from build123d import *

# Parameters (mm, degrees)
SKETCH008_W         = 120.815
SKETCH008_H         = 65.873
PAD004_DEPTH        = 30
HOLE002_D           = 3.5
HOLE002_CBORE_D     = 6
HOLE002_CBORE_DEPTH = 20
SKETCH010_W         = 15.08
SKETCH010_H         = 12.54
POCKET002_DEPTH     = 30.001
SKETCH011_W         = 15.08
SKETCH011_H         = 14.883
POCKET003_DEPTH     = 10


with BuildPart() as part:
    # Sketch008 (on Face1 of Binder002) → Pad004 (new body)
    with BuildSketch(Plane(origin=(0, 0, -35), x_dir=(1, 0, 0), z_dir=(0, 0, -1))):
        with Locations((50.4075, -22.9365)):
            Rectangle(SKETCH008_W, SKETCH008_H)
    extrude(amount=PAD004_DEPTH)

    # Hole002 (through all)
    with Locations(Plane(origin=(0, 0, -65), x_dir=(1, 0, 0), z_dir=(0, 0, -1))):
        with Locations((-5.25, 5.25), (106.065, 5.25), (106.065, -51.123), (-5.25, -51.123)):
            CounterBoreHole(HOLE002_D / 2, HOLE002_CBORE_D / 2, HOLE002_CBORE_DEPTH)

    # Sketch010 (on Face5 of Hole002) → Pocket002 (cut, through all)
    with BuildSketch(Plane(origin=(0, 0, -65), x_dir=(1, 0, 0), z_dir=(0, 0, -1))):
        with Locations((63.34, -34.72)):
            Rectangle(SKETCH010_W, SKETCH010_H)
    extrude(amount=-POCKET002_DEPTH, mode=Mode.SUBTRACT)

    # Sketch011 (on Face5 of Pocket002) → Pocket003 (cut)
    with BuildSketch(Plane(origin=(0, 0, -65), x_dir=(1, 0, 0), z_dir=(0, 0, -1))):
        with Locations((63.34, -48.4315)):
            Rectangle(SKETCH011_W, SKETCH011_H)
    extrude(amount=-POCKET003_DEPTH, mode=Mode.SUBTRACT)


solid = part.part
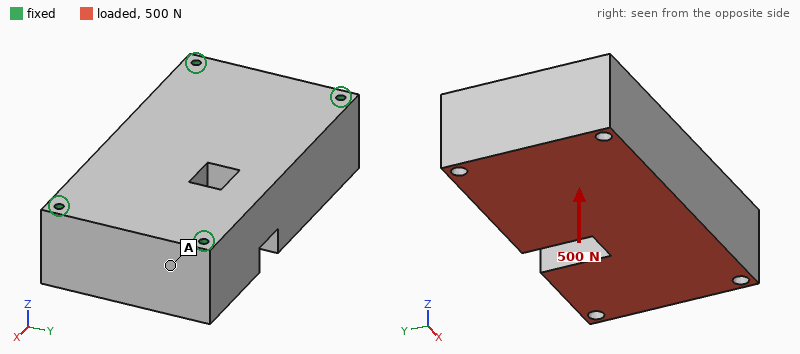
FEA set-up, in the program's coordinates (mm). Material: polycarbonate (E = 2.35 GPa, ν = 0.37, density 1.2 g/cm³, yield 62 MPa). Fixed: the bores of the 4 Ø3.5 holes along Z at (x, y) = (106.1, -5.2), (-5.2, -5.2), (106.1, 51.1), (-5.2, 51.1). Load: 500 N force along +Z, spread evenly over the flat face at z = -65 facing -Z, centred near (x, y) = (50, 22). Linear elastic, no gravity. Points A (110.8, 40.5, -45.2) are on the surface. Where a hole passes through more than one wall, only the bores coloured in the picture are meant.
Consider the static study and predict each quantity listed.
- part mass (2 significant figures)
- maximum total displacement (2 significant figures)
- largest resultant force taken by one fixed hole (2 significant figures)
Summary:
270 g
31 µm
160 N
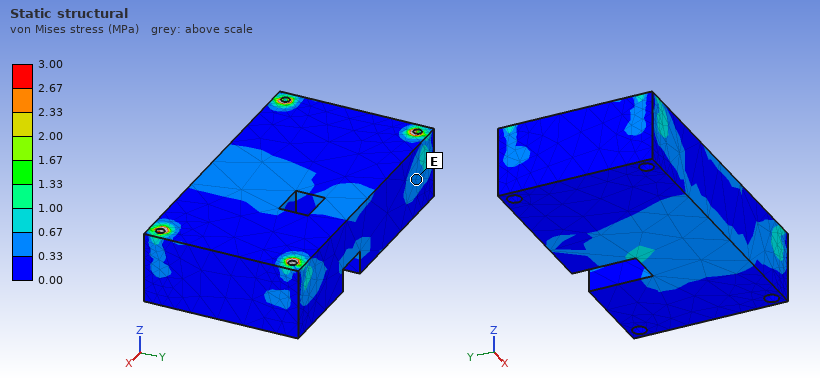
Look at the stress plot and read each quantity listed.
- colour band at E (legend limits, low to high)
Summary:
0.33 to 0.67 MPa
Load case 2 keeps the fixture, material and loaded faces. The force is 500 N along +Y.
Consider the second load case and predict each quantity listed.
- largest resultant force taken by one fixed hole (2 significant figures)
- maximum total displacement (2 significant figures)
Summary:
190 N
23 µm
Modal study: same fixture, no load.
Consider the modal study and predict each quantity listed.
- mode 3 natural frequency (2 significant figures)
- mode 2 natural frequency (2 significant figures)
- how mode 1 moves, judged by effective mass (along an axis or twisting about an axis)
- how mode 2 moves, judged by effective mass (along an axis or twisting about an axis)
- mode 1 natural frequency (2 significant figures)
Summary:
2400 Hz
2200 Hz
along Z
along Y
1400 Hz
